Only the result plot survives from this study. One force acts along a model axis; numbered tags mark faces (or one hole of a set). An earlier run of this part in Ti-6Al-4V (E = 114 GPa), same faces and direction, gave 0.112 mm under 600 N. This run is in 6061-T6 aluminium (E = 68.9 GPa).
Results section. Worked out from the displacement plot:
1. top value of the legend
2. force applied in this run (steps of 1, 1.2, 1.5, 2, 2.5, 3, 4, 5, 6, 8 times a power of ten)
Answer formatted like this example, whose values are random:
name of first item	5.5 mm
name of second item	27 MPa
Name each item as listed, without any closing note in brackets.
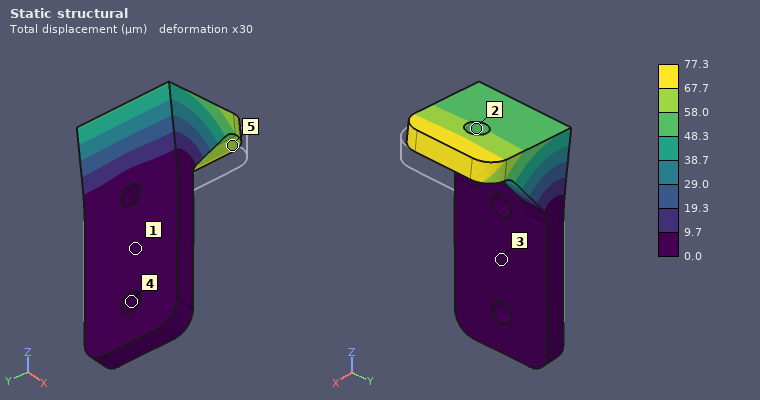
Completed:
top value of the legend	77.3 µm
force applied in this run	250 N
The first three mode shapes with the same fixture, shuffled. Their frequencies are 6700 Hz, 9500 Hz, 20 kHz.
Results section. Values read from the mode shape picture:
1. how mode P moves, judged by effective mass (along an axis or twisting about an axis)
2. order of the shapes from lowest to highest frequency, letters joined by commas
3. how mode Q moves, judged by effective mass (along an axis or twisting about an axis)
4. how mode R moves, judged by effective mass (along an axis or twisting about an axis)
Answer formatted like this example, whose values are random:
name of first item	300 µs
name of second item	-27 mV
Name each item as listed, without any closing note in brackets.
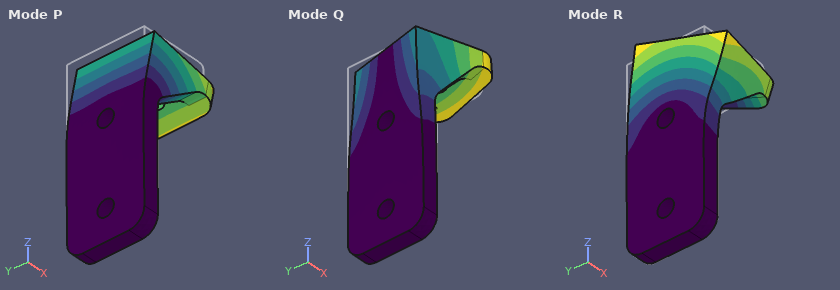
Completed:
how mode P moves, judged by effective mass	along X
order of the shapes from lowest to highest frequency, letters joined by commas	P, Q, R
how mode Q moves, judged by effective mass	along Y
how mode R moves, judged by effective mass	along Y
